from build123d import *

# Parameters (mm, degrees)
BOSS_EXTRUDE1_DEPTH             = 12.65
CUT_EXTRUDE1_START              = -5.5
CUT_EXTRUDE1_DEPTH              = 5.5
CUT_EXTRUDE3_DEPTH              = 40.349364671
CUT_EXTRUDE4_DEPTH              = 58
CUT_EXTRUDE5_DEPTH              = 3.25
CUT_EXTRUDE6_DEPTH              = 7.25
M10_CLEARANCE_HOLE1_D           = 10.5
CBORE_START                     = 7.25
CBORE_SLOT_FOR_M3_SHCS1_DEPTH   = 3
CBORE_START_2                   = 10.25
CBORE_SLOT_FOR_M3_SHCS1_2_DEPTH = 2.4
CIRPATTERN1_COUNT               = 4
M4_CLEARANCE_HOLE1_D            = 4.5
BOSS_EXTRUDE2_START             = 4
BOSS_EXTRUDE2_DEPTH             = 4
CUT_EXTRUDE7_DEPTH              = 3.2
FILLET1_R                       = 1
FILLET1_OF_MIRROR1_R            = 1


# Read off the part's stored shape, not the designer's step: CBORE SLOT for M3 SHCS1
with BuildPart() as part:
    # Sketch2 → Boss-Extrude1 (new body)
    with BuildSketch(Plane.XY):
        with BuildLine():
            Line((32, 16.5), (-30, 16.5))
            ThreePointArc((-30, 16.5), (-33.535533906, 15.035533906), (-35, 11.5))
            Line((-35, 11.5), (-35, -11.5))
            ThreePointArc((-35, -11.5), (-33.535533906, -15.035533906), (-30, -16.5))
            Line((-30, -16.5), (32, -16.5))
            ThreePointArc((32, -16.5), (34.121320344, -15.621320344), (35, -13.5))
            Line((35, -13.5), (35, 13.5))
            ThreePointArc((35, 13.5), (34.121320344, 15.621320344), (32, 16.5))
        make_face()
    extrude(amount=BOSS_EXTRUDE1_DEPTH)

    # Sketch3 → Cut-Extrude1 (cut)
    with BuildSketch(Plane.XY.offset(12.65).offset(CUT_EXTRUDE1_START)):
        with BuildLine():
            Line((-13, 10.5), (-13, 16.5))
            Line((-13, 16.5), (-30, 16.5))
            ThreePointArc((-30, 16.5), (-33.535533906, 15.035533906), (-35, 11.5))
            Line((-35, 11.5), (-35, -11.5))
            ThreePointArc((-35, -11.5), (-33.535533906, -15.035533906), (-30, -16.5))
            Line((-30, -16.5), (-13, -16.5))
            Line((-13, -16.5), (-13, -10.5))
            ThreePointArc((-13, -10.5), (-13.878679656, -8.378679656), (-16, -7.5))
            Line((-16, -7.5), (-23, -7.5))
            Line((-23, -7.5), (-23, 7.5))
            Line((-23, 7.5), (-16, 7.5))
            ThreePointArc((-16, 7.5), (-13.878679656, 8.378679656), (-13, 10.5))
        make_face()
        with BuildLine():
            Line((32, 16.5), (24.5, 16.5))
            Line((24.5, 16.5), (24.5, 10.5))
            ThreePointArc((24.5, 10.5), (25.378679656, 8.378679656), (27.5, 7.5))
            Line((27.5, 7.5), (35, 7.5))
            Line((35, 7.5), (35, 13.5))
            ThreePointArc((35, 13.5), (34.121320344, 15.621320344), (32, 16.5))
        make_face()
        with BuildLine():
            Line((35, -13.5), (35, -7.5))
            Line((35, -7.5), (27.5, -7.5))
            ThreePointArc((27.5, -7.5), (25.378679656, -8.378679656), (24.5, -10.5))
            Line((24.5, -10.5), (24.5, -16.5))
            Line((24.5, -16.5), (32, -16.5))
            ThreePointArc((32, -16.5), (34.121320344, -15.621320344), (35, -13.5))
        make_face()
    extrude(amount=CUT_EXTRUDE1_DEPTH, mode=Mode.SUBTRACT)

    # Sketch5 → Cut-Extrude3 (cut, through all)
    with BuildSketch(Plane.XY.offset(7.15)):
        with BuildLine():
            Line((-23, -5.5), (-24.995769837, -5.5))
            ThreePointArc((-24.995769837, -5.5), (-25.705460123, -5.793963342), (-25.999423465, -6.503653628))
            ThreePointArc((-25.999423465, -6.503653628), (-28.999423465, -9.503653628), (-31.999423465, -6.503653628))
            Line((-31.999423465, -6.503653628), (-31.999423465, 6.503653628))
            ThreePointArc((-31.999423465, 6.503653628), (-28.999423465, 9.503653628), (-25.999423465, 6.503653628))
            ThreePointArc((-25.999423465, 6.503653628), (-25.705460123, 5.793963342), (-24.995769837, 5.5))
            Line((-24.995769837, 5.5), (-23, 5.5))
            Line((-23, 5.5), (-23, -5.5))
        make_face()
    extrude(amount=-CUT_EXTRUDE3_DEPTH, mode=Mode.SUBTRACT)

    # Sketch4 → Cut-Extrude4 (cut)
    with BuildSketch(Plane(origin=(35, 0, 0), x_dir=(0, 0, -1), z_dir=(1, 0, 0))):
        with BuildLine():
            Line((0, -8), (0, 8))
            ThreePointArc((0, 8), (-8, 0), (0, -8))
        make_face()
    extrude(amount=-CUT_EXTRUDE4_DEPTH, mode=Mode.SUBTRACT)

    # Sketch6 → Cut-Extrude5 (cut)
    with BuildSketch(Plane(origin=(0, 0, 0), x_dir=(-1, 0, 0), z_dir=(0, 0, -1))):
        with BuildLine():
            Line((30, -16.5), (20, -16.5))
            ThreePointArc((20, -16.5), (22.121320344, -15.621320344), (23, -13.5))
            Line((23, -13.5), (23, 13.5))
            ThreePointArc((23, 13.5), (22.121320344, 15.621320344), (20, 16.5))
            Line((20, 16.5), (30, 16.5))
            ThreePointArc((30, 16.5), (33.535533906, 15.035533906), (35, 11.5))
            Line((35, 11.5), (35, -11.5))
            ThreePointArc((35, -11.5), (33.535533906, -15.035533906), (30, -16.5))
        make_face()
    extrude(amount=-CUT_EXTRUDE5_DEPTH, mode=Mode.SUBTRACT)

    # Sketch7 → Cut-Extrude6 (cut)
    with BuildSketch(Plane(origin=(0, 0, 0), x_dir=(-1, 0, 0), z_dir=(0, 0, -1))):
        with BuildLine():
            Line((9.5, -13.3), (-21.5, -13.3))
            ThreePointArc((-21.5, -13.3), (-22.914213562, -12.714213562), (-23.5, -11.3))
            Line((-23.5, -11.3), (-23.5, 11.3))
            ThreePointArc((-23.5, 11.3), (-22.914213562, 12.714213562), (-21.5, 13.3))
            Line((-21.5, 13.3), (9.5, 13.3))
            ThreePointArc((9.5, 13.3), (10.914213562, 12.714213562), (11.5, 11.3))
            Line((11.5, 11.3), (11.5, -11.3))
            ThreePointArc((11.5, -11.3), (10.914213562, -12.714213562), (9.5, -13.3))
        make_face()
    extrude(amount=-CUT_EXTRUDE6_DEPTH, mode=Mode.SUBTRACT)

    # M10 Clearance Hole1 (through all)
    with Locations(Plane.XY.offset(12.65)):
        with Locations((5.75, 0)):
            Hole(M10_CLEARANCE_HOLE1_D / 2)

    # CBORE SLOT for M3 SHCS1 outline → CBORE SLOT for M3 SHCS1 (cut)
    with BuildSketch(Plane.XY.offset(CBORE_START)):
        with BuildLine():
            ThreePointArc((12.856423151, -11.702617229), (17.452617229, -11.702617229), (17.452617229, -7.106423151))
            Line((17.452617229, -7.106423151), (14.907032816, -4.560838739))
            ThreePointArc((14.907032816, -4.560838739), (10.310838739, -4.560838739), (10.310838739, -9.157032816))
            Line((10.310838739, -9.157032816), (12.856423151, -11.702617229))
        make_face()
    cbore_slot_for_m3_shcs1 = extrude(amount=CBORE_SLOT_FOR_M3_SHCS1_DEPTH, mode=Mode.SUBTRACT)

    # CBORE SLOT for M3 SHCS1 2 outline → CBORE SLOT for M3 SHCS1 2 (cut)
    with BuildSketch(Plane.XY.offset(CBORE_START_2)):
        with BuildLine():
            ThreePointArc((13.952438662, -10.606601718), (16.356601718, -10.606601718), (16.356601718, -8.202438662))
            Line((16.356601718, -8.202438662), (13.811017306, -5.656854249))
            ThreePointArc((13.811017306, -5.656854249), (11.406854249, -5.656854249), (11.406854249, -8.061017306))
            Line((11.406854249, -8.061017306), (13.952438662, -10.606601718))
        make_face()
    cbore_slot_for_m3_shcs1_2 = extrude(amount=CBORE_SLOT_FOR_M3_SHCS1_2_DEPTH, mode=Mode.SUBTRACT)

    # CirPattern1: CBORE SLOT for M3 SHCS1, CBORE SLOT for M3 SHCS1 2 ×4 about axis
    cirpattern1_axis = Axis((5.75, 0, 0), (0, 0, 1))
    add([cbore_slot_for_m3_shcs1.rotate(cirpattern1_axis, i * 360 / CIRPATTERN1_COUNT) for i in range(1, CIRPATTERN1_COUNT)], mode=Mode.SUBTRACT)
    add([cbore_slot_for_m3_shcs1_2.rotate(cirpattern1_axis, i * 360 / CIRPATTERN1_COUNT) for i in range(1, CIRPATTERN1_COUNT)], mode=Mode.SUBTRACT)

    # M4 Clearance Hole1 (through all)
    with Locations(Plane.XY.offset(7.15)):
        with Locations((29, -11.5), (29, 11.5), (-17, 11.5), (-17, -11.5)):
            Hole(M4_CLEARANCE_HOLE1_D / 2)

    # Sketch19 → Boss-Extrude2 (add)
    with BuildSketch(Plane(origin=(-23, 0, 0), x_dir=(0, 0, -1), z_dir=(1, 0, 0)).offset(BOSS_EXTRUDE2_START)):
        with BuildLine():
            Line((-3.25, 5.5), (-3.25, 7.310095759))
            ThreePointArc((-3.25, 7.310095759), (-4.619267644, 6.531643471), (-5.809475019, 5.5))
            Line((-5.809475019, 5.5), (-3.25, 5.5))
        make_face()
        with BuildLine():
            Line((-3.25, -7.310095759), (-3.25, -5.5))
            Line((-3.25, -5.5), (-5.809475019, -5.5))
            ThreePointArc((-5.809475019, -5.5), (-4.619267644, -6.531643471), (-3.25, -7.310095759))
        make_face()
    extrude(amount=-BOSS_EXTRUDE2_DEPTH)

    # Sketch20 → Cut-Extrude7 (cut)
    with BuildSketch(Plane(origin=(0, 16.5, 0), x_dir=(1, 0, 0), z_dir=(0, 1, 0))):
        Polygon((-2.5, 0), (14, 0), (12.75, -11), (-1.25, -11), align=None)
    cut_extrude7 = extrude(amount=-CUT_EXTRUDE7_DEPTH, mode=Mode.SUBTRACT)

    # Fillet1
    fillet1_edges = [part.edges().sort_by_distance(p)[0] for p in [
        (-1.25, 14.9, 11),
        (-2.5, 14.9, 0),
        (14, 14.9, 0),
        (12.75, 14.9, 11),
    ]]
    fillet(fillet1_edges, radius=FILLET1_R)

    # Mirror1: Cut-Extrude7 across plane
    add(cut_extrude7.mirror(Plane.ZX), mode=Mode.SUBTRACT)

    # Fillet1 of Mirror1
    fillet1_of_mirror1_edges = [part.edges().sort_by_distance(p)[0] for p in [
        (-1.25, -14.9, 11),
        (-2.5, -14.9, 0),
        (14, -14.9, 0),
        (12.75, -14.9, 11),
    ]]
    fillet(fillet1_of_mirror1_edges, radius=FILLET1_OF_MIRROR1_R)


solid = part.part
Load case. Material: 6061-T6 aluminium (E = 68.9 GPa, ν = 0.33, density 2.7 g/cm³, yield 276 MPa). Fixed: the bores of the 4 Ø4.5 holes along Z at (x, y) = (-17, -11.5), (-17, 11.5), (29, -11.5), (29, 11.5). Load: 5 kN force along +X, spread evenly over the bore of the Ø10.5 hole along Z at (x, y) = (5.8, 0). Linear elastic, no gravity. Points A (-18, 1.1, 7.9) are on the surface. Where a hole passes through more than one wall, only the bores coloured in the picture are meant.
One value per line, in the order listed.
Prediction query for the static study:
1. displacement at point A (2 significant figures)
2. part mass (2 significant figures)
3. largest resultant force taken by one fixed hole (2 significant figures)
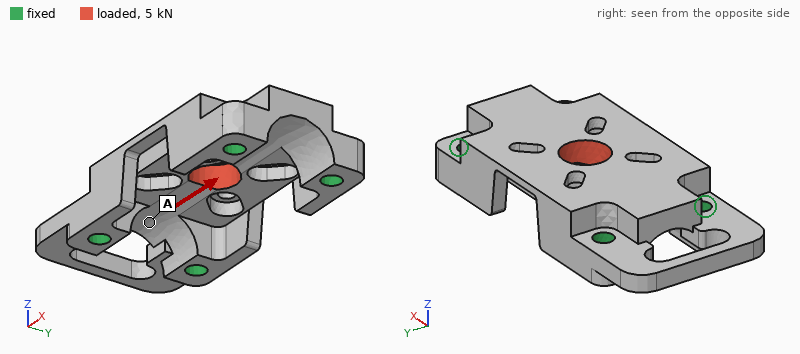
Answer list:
6.3 µm
30 g
1.3 kN
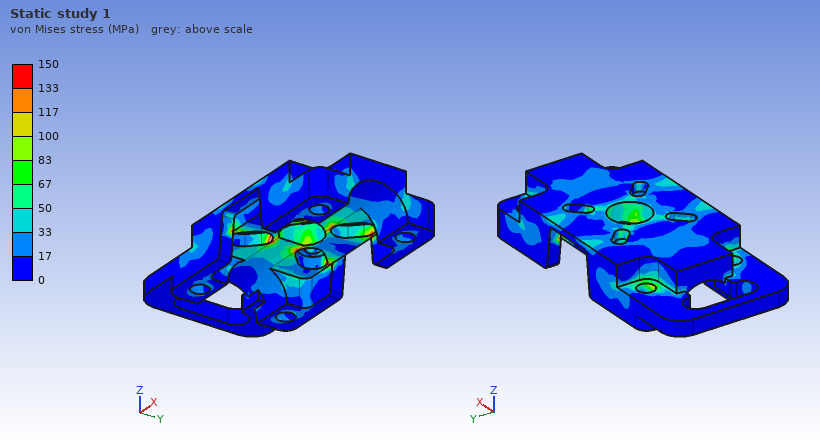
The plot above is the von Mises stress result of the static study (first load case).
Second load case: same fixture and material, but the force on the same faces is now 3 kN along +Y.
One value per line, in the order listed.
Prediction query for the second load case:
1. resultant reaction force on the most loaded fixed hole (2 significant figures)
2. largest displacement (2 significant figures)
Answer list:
1000 N
22 µm
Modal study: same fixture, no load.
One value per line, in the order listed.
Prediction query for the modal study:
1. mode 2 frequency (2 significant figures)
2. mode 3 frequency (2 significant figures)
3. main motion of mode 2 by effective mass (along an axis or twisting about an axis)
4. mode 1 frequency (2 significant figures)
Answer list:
16 kHz
19 kHz
along Z
12 kHz
